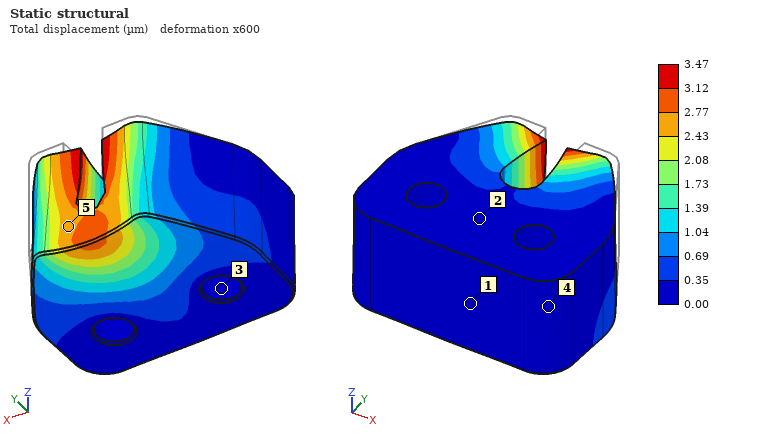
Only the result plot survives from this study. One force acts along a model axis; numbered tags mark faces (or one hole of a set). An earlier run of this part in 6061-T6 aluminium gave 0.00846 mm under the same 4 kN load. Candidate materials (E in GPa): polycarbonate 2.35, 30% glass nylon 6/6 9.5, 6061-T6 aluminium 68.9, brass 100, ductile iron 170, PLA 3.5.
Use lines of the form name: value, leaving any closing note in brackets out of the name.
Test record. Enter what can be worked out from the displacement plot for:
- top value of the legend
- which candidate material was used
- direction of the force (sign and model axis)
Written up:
top value of the legend: 3.47 µm
which candidate material was used: ductile iron
direction of the force: -Y
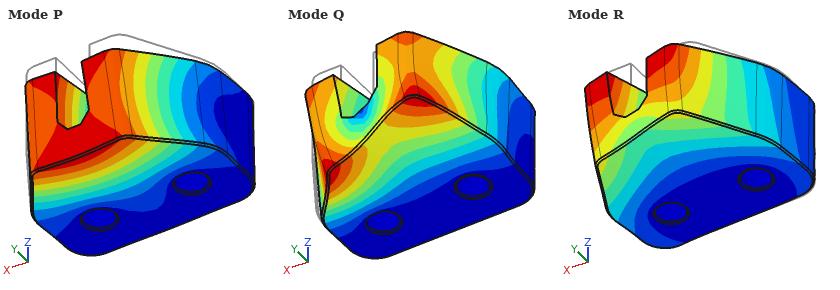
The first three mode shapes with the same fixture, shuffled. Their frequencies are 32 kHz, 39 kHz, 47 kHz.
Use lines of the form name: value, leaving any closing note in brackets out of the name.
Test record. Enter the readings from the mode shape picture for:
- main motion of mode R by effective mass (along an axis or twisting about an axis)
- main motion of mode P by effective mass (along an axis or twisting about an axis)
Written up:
main motion of mode R by effective mass: along X
main motion of mode P by effective mass: along Z
